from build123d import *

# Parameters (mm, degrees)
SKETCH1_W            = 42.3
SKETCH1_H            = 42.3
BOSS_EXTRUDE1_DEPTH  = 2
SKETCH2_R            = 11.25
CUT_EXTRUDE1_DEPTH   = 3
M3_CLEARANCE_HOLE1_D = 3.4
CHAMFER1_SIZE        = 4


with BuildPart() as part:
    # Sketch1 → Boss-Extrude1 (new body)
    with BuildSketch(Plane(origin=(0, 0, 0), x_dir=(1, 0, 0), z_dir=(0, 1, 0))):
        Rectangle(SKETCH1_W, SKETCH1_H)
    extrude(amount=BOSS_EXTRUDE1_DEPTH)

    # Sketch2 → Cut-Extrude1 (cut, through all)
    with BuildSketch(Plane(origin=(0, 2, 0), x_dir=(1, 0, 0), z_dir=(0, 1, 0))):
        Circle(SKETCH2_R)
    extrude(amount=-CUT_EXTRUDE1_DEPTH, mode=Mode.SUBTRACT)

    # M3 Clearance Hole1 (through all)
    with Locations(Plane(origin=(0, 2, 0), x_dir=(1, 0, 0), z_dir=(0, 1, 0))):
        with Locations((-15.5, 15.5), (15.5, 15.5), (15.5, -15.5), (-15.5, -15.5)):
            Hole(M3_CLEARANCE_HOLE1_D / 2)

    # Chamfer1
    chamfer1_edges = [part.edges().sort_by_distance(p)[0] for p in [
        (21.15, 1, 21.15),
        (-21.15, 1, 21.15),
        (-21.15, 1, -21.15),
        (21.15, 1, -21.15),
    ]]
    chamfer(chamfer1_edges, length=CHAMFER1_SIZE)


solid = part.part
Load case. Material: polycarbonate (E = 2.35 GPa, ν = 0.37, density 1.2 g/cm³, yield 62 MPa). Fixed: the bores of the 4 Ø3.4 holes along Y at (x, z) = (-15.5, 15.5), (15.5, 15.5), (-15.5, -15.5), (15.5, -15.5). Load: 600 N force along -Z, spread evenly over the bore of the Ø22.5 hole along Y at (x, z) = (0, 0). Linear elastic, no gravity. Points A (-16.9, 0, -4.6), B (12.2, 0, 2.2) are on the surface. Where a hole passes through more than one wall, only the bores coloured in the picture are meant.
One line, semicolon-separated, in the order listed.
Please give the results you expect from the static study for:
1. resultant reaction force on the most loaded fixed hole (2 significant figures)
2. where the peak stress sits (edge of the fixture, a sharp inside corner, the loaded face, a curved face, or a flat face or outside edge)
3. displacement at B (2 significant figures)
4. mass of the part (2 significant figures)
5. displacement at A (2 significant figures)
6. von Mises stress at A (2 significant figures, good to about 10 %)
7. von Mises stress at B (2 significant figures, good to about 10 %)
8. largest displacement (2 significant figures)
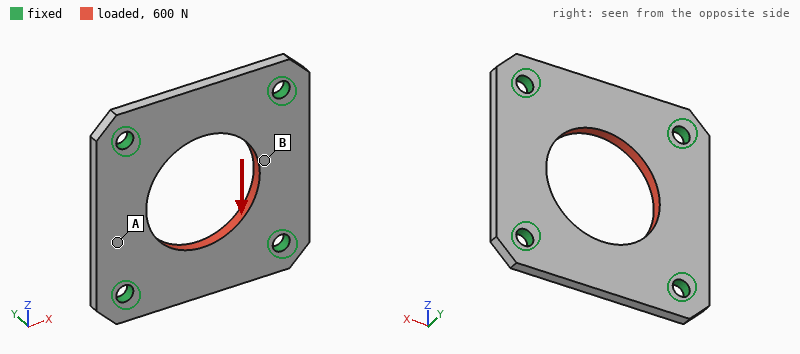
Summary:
150 N; edge of the fixture; 32 µm; 3.2 g; 20 µm; 4.3 MPa; 7.5 MPa; 83 µm
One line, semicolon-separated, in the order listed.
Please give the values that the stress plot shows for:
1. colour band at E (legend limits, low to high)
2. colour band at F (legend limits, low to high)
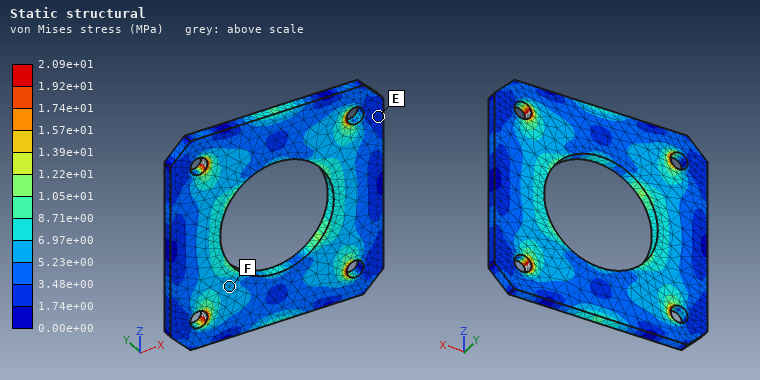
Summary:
1.74e+00 to 3.48e+00 MPa; 5.23e+00 to 6.97e+00 MPa
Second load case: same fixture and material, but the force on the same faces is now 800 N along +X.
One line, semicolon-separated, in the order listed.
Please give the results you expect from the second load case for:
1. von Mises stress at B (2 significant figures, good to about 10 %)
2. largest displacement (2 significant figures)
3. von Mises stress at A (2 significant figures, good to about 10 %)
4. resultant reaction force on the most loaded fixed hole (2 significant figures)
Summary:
5.8 MPa; 0.11 mm; 5.9 MPa; 210 N
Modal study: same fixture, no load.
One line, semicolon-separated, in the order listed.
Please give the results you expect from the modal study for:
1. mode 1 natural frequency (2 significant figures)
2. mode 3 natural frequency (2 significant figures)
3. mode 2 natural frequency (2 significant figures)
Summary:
3300 Hz; 3500 Hz; 3400 Hz
